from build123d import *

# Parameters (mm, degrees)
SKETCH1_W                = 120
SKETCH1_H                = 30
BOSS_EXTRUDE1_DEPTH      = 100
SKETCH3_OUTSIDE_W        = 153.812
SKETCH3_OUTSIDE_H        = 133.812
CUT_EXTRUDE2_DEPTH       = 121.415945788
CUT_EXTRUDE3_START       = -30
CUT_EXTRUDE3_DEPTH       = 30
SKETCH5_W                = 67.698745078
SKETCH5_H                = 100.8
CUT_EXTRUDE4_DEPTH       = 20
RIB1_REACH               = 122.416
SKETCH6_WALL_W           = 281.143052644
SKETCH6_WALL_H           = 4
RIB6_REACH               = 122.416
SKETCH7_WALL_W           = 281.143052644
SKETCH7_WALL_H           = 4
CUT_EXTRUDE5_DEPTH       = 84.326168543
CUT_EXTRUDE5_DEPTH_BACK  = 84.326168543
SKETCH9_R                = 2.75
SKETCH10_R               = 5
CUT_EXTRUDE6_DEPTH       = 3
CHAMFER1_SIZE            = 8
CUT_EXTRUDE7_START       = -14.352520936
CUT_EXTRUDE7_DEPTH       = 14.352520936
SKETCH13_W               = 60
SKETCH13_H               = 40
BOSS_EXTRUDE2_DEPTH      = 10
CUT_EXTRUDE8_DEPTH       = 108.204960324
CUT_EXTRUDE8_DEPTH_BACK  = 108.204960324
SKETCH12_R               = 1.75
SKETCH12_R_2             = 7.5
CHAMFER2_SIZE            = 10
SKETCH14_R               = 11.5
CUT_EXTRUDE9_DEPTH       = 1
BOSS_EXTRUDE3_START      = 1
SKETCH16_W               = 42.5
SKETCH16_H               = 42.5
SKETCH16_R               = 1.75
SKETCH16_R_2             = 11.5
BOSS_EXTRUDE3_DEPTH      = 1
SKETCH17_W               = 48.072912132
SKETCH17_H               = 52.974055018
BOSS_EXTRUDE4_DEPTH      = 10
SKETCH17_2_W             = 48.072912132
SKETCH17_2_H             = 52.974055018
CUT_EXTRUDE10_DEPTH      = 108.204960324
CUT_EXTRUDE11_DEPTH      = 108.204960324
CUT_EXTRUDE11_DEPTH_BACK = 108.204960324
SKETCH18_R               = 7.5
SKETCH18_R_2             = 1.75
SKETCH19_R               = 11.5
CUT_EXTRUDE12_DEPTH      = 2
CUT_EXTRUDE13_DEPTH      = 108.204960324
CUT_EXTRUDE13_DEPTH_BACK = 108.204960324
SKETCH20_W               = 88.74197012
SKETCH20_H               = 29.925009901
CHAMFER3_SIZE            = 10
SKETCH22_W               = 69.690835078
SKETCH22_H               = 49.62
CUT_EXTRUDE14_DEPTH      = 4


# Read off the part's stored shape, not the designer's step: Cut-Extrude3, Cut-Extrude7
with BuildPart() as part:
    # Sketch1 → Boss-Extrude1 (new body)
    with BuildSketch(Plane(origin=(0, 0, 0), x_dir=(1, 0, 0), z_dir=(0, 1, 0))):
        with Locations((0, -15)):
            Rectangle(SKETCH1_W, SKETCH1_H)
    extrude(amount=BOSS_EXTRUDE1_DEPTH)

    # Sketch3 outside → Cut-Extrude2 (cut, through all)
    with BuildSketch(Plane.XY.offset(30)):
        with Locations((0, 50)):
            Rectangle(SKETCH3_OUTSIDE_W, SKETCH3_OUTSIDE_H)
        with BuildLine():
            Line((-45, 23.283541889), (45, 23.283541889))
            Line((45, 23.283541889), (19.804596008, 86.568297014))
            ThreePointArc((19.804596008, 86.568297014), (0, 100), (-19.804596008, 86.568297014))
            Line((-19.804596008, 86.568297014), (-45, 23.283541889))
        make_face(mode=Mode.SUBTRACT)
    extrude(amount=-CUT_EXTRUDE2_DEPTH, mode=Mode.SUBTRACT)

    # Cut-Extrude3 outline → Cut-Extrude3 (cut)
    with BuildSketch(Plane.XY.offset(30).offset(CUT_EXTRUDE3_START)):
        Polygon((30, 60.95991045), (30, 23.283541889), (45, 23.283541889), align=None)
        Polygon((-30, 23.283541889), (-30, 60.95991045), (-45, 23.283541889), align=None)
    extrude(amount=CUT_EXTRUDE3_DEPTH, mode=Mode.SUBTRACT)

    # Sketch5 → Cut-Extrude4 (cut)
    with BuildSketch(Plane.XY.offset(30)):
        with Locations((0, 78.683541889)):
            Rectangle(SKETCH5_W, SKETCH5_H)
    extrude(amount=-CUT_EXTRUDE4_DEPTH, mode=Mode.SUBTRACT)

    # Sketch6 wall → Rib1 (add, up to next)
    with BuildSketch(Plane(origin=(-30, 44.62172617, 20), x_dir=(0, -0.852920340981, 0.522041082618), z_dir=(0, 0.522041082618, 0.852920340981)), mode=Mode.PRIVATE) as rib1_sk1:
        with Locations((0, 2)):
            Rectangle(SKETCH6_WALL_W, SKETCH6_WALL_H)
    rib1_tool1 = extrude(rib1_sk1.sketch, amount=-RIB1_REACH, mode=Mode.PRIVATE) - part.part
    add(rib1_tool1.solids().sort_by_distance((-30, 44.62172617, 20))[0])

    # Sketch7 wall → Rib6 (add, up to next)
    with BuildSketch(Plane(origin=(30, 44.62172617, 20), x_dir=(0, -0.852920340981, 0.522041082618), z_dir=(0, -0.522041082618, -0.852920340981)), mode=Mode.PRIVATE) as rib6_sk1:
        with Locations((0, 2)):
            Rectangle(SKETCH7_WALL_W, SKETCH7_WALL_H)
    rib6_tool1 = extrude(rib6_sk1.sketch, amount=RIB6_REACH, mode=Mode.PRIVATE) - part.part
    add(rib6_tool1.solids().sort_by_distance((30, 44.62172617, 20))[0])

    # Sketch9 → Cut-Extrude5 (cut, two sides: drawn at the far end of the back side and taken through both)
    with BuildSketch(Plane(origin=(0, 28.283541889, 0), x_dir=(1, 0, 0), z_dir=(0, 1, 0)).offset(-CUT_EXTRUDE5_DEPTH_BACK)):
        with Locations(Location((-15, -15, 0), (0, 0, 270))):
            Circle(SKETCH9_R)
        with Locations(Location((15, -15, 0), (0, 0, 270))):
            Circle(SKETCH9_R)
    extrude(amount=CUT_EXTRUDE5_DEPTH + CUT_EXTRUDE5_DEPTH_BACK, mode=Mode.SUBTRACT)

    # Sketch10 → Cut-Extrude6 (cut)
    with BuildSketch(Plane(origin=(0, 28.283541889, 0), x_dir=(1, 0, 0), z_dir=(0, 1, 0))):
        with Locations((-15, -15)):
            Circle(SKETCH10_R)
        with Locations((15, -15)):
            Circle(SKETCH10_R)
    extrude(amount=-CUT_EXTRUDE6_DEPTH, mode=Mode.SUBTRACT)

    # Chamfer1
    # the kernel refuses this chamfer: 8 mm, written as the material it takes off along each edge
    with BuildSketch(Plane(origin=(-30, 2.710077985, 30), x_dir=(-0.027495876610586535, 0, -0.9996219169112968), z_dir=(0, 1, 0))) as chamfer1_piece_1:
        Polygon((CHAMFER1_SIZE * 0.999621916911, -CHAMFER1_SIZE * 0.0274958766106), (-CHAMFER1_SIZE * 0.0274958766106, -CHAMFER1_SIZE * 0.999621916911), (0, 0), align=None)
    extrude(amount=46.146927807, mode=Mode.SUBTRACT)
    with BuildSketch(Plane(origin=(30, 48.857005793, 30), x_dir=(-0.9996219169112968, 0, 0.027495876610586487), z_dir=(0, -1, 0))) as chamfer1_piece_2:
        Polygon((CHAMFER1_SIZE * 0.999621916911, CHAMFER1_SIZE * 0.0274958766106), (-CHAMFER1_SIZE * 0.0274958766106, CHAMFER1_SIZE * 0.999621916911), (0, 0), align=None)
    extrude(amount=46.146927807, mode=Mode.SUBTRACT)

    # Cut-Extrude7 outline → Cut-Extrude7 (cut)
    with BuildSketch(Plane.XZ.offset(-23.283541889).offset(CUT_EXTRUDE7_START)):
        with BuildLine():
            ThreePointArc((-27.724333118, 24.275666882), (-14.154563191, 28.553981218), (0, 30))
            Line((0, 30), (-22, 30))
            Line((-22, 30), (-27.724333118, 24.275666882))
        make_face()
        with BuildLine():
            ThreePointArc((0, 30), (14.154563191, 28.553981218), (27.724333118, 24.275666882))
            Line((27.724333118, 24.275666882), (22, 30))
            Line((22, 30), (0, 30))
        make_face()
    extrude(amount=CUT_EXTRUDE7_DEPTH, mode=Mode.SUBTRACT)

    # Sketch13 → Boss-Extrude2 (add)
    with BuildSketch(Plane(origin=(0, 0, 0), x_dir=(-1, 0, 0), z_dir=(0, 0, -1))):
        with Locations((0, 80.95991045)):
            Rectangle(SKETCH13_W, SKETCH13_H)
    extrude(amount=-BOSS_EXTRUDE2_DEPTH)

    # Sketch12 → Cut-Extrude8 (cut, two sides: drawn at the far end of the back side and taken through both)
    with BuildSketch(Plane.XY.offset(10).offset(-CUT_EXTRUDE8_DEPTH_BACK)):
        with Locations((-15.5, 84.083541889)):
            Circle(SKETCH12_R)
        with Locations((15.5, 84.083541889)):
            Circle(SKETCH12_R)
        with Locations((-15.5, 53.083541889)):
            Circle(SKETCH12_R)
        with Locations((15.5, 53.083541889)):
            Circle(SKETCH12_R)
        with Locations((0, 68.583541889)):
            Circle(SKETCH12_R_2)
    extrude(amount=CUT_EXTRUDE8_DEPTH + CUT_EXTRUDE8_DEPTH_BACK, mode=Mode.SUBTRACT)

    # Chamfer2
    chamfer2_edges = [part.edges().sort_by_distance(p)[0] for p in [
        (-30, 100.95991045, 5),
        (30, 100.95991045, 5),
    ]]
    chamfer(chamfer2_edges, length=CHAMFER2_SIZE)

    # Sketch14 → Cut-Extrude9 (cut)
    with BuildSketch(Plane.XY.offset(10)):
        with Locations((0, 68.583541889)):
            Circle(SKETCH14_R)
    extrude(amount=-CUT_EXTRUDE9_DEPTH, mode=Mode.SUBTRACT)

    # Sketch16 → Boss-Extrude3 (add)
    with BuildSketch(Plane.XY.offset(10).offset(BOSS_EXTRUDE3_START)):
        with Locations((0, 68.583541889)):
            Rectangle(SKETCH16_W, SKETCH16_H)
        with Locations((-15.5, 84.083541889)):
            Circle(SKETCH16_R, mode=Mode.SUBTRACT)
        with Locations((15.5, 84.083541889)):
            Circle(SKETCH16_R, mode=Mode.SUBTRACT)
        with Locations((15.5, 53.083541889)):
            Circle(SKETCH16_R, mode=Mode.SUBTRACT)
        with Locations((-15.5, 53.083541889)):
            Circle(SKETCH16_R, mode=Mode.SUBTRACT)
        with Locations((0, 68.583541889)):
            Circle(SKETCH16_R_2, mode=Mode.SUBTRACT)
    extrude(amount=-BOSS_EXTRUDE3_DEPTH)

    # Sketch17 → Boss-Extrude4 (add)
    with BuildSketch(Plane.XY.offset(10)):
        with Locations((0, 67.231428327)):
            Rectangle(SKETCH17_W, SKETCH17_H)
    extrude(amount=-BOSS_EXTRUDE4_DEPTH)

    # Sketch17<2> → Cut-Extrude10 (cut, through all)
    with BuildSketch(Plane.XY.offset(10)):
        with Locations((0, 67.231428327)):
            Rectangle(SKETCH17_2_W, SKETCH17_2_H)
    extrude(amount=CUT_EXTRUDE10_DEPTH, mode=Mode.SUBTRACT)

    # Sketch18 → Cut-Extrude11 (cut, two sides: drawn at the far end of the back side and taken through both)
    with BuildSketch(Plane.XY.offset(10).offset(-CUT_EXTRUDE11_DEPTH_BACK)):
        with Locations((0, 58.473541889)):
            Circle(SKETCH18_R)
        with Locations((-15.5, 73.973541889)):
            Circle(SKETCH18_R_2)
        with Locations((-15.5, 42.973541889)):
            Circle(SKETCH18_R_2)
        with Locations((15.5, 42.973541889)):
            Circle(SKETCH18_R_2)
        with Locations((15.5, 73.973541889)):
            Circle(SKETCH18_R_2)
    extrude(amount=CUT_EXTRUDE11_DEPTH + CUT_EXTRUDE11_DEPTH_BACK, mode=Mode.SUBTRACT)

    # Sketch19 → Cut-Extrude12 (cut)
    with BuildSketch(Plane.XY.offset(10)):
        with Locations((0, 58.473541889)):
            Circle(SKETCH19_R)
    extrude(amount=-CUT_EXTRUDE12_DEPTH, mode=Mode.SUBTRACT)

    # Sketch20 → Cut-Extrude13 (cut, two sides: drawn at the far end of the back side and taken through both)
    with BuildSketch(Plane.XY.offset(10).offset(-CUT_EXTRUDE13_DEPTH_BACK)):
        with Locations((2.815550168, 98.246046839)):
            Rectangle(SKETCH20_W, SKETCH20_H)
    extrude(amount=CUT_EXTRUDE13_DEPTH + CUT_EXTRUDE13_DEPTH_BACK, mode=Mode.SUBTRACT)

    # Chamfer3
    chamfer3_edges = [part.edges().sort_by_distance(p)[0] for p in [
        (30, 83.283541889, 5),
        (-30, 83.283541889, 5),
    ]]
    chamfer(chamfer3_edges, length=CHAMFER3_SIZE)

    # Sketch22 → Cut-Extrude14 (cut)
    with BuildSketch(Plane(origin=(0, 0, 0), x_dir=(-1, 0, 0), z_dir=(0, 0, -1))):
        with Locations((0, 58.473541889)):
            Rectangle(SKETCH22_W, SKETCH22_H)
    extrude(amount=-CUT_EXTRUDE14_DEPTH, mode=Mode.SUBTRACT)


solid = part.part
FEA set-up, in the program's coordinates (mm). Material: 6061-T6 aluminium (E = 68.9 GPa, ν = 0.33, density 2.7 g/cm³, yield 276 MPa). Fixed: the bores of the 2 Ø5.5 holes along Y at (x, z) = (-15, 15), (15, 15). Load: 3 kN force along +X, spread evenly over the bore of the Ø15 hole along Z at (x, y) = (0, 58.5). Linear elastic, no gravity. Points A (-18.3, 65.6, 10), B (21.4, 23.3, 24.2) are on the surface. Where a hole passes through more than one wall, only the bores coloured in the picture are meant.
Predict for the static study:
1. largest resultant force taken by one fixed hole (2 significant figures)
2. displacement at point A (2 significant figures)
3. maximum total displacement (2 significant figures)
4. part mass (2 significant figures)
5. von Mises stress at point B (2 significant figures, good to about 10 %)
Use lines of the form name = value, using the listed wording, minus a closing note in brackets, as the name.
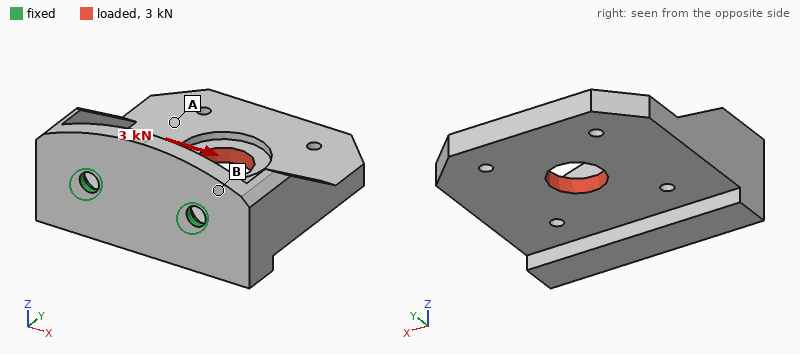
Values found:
largest resultant force taken by one fixed hole = 3.6 kN
displacement at point A = 0.15 mm
maximum total displacement = 0.21 mm
part mass = 78 g
von Mises stress at point B = 45 MPa
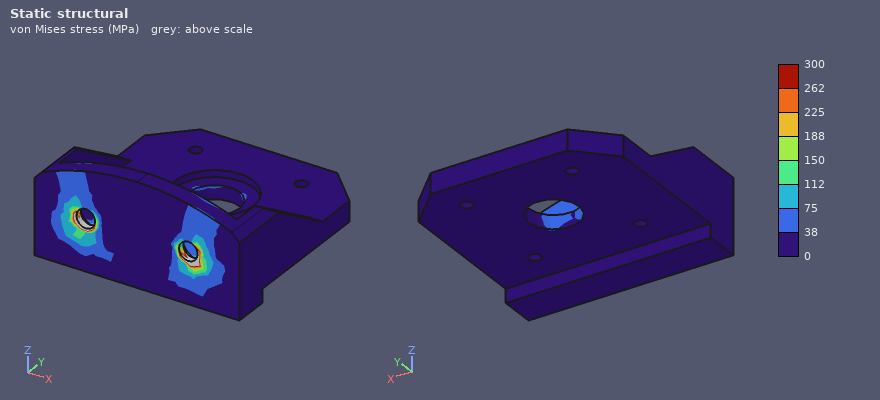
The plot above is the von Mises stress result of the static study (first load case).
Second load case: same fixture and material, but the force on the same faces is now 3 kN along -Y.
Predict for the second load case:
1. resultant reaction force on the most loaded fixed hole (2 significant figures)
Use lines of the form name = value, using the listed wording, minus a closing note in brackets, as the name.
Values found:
resultant reaction force on the most loaded fixed hole = 1.5 kN
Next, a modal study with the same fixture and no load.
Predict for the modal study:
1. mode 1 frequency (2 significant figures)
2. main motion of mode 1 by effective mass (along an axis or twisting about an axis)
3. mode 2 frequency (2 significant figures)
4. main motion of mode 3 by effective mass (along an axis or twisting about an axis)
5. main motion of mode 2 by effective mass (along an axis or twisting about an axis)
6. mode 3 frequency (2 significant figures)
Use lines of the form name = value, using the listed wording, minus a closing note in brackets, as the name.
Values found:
mode 1 frequency = 1000 Hz
main motion of mode 1 by effective mass = along Z
mode 2 frequency = 2800 Hz
main motion of mode 3 by effective mass = along X
main motion of mode 2 by effective mass = along X
mode 3 frequency = 4300 Hz
